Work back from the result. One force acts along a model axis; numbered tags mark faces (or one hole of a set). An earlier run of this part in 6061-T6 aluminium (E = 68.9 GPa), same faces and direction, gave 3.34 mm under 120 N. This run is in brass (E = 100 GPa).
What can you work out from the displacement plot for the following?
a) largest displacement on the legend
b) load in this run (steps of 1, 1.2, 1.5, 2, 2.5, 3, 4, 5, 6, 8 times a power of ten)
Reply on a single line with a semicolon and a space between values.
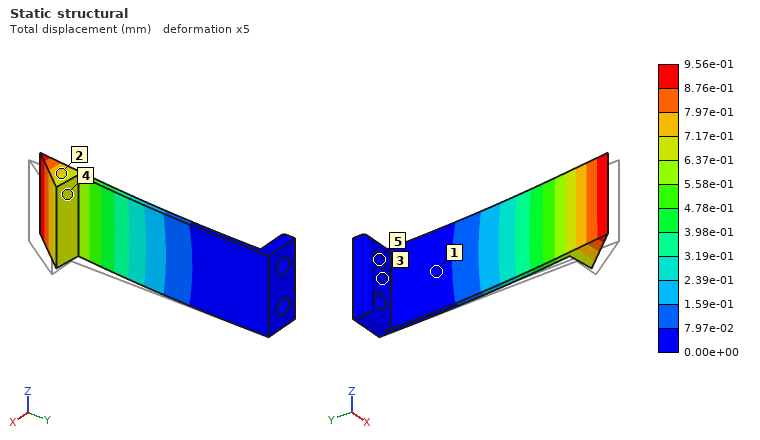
9.56e-01 mm; 50 N
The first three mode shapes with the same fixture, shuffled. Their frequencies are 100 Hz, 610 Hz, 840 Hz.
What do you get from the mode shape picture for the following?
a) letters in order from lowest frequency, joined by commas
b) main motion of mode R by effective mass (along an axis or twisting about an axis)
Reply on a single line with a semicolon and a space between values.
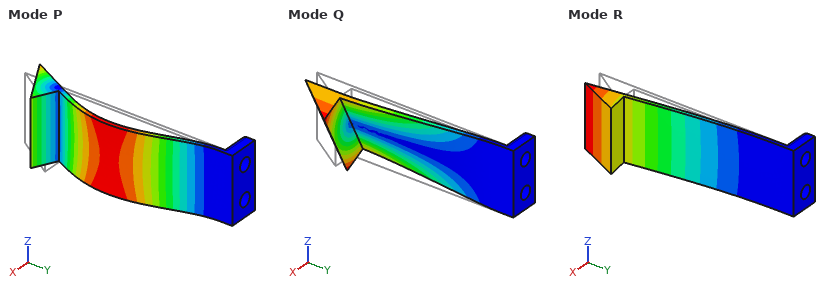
R, Q, P; along X
